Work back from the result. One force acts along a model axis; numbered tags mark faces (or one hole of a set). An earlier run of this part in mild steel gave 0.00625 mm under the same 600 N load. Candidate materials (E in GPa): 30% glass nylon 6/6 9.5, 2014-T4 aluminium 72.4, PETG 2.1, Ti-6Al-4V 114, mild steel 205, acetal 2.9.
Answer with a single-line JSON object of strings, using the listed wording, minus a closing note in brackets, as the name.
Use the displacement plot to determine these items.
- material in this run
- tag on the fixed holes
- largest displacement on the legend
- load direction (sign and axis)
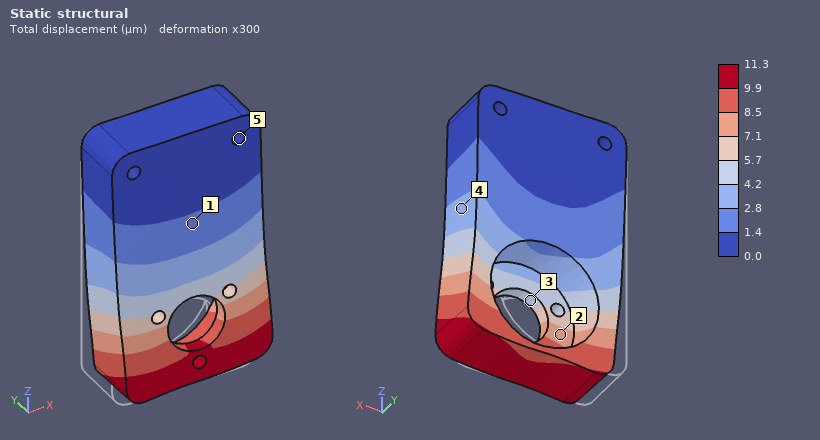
{"material in this run": "Ti-6Al-4V", "tag on the fixed holes": "5", "largest displacement on the legend": "11.3 µm", "load direction": "+X"}
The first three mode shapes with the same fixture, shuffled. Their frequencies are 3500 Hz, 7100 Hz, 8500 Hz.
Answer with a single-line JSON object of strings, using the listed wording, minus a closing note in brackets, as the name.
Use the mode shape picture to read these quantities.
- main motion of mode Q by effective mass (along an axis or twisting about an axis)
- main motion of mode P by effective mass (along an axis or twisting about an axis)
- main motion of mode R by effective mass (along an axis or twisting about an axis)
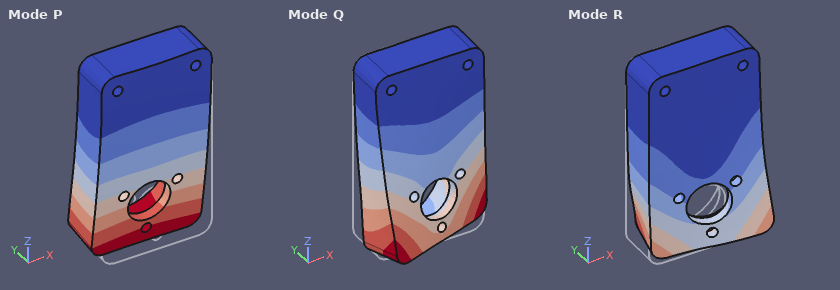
{"main motion of mode Q by effective mass": "along X", "main motion of mode P by effective mass": "along Y", "main motion of mode R by effective mass": "along X"}
